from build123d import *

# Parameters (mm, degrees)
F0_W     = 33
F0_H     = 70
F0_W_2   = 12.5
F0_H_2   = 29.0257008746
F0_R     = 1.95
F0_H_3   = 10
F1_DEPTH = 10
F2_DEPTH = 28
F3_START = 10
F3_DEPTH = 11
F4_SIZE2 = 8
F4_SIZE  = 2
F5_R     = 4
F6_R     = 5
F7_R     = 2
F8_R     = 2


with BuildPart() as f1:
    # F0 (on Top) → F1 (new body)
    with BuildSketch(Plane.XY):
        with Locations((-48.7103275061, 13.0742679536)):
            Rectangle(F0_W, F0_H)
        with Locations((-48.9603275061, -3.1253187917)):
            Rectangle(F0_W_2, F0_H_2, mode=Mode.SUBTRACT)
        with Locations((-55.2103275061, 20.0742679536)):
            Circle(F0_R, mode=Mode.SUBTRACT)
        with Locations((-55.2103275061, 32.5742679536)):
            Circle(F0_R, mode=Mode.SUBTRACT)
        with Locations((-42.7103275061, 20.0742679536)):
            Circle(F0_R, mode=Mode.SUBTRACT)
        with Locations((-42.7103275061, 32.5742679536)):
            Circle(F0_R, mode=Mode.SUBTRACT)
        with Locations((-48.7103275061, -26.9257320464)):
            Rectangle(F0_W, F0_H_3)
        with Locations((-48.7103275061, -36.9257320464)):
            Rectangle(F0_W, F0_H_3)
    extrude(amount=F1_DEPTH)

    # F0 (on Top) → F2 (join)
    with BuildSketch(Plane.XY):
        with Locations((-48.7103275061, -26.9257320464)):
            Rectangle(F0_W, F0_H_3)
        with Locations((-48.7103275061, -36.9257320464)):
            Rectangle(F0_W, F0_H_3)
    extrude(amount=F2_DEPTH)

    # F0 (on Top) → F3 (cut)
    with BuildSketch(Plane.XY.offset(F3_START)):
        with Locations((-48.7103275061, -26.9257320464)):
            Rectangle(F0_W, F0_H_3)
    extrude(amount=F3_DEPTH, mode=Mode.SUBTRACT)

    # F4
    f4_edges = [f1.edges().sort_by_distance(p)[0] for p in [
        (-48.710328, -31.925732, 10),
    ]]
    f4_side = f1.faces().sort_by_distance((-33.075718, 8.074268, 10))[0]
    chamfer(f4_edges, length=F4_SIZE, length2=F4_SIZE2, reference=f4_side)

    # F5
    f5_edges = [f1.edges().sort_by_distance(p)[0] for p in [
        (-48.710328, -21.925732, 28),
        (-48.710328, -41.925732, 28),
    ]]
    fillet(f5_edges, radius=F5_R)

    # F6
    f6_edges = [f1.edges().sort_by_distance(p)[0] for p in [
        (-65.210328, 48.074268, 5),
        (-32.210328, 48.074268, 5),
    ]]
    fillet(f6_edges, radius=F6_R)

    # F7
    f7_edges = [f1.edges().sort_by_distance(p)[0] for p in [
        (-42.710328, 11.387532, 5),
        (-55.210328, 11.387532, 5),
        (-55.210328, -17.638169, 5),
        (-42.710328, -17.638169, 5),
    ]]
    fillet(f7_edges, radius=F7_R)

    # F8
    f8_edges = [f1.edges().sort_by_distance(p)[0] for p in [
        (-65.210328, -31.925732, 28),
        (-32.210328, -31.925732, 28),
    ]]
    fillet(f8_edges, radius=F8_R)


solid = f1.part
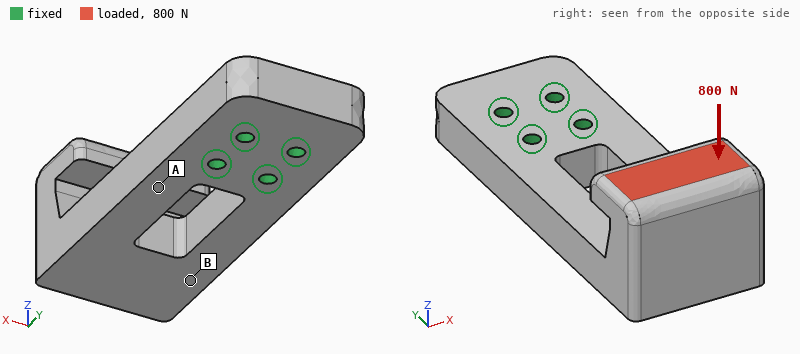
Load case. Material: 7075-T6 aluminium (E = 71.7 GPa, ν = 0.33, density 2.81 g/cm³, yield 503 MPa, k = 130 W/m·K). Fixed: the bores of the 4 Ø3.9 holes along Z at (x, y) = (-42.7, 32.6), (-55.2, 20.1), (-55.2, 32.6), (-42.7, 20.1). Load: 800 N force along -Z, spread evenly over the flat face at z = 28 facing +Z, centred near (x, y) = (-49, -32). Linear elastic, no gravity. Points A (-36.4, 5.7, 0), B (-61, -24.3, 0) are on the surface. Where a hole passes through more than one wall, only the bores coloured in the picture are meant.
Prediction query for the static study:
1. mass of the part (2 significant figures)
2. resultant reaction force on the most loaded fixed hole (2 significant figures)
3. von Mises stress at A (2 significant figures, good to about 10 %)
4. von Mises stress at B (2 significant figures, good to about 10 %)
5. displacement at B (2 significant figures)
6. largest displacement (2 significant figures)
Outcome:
95 g
840 N
85 MPa
15 MPa
0.23 mm
0.41 mm
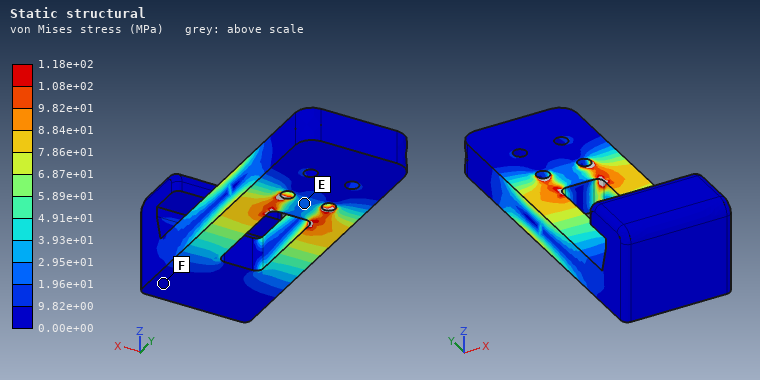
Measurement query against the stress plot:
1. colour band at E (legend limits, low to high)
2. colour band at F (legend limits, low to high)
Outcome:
1.96e+01 to 2.95e+01 MPa
0.00e+00 to 9.82e+00 MPa
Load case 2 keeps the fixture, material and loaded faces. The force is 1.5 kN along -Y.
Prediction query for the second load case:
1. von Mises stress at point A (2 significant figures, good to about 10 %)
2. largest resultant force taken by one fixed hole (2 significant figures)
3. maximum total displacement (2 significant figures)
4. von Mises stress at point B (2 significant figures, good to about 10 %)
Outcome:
92 MPa
690 N
0.58 mm
67 MPa
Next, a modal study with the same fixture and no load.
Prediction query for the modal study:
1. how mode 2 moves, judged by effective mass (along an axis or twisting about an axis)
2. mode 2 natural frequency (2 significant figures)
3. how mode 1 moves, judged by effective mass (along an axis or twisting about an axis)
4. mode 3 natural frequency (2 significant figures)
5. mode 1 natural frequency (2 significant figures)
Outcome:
along X
2200 Hz
along Z
3700 Hz
1100 Hz
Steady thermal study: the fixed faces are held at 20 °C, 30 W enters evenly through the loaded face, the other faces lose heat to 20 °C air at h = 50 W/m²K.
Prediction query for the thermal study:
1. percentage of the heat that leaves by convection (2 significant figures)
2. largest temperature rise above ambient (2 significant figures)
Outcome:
35 %
51 K
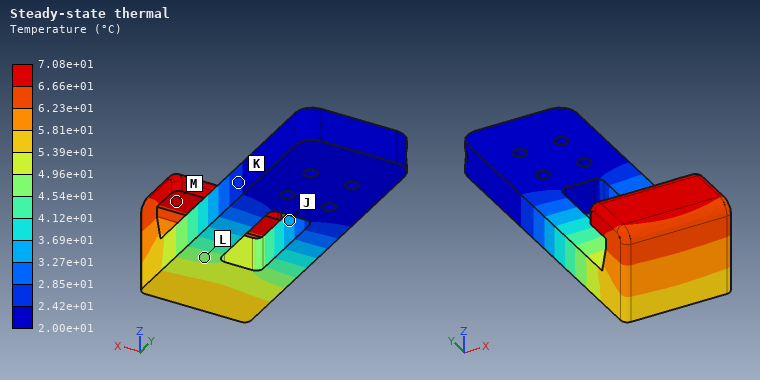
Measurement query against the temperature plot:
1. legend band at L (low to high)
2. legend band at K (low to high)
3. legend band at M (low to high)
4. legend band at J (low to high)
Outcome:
4.54e+01 to 4.96e+01 °C
2.42e+01 to 2.85e+01 °C
6.66e+01 to 7.08e+01 °C
3.27e+01 to 3.69e+01 °C
